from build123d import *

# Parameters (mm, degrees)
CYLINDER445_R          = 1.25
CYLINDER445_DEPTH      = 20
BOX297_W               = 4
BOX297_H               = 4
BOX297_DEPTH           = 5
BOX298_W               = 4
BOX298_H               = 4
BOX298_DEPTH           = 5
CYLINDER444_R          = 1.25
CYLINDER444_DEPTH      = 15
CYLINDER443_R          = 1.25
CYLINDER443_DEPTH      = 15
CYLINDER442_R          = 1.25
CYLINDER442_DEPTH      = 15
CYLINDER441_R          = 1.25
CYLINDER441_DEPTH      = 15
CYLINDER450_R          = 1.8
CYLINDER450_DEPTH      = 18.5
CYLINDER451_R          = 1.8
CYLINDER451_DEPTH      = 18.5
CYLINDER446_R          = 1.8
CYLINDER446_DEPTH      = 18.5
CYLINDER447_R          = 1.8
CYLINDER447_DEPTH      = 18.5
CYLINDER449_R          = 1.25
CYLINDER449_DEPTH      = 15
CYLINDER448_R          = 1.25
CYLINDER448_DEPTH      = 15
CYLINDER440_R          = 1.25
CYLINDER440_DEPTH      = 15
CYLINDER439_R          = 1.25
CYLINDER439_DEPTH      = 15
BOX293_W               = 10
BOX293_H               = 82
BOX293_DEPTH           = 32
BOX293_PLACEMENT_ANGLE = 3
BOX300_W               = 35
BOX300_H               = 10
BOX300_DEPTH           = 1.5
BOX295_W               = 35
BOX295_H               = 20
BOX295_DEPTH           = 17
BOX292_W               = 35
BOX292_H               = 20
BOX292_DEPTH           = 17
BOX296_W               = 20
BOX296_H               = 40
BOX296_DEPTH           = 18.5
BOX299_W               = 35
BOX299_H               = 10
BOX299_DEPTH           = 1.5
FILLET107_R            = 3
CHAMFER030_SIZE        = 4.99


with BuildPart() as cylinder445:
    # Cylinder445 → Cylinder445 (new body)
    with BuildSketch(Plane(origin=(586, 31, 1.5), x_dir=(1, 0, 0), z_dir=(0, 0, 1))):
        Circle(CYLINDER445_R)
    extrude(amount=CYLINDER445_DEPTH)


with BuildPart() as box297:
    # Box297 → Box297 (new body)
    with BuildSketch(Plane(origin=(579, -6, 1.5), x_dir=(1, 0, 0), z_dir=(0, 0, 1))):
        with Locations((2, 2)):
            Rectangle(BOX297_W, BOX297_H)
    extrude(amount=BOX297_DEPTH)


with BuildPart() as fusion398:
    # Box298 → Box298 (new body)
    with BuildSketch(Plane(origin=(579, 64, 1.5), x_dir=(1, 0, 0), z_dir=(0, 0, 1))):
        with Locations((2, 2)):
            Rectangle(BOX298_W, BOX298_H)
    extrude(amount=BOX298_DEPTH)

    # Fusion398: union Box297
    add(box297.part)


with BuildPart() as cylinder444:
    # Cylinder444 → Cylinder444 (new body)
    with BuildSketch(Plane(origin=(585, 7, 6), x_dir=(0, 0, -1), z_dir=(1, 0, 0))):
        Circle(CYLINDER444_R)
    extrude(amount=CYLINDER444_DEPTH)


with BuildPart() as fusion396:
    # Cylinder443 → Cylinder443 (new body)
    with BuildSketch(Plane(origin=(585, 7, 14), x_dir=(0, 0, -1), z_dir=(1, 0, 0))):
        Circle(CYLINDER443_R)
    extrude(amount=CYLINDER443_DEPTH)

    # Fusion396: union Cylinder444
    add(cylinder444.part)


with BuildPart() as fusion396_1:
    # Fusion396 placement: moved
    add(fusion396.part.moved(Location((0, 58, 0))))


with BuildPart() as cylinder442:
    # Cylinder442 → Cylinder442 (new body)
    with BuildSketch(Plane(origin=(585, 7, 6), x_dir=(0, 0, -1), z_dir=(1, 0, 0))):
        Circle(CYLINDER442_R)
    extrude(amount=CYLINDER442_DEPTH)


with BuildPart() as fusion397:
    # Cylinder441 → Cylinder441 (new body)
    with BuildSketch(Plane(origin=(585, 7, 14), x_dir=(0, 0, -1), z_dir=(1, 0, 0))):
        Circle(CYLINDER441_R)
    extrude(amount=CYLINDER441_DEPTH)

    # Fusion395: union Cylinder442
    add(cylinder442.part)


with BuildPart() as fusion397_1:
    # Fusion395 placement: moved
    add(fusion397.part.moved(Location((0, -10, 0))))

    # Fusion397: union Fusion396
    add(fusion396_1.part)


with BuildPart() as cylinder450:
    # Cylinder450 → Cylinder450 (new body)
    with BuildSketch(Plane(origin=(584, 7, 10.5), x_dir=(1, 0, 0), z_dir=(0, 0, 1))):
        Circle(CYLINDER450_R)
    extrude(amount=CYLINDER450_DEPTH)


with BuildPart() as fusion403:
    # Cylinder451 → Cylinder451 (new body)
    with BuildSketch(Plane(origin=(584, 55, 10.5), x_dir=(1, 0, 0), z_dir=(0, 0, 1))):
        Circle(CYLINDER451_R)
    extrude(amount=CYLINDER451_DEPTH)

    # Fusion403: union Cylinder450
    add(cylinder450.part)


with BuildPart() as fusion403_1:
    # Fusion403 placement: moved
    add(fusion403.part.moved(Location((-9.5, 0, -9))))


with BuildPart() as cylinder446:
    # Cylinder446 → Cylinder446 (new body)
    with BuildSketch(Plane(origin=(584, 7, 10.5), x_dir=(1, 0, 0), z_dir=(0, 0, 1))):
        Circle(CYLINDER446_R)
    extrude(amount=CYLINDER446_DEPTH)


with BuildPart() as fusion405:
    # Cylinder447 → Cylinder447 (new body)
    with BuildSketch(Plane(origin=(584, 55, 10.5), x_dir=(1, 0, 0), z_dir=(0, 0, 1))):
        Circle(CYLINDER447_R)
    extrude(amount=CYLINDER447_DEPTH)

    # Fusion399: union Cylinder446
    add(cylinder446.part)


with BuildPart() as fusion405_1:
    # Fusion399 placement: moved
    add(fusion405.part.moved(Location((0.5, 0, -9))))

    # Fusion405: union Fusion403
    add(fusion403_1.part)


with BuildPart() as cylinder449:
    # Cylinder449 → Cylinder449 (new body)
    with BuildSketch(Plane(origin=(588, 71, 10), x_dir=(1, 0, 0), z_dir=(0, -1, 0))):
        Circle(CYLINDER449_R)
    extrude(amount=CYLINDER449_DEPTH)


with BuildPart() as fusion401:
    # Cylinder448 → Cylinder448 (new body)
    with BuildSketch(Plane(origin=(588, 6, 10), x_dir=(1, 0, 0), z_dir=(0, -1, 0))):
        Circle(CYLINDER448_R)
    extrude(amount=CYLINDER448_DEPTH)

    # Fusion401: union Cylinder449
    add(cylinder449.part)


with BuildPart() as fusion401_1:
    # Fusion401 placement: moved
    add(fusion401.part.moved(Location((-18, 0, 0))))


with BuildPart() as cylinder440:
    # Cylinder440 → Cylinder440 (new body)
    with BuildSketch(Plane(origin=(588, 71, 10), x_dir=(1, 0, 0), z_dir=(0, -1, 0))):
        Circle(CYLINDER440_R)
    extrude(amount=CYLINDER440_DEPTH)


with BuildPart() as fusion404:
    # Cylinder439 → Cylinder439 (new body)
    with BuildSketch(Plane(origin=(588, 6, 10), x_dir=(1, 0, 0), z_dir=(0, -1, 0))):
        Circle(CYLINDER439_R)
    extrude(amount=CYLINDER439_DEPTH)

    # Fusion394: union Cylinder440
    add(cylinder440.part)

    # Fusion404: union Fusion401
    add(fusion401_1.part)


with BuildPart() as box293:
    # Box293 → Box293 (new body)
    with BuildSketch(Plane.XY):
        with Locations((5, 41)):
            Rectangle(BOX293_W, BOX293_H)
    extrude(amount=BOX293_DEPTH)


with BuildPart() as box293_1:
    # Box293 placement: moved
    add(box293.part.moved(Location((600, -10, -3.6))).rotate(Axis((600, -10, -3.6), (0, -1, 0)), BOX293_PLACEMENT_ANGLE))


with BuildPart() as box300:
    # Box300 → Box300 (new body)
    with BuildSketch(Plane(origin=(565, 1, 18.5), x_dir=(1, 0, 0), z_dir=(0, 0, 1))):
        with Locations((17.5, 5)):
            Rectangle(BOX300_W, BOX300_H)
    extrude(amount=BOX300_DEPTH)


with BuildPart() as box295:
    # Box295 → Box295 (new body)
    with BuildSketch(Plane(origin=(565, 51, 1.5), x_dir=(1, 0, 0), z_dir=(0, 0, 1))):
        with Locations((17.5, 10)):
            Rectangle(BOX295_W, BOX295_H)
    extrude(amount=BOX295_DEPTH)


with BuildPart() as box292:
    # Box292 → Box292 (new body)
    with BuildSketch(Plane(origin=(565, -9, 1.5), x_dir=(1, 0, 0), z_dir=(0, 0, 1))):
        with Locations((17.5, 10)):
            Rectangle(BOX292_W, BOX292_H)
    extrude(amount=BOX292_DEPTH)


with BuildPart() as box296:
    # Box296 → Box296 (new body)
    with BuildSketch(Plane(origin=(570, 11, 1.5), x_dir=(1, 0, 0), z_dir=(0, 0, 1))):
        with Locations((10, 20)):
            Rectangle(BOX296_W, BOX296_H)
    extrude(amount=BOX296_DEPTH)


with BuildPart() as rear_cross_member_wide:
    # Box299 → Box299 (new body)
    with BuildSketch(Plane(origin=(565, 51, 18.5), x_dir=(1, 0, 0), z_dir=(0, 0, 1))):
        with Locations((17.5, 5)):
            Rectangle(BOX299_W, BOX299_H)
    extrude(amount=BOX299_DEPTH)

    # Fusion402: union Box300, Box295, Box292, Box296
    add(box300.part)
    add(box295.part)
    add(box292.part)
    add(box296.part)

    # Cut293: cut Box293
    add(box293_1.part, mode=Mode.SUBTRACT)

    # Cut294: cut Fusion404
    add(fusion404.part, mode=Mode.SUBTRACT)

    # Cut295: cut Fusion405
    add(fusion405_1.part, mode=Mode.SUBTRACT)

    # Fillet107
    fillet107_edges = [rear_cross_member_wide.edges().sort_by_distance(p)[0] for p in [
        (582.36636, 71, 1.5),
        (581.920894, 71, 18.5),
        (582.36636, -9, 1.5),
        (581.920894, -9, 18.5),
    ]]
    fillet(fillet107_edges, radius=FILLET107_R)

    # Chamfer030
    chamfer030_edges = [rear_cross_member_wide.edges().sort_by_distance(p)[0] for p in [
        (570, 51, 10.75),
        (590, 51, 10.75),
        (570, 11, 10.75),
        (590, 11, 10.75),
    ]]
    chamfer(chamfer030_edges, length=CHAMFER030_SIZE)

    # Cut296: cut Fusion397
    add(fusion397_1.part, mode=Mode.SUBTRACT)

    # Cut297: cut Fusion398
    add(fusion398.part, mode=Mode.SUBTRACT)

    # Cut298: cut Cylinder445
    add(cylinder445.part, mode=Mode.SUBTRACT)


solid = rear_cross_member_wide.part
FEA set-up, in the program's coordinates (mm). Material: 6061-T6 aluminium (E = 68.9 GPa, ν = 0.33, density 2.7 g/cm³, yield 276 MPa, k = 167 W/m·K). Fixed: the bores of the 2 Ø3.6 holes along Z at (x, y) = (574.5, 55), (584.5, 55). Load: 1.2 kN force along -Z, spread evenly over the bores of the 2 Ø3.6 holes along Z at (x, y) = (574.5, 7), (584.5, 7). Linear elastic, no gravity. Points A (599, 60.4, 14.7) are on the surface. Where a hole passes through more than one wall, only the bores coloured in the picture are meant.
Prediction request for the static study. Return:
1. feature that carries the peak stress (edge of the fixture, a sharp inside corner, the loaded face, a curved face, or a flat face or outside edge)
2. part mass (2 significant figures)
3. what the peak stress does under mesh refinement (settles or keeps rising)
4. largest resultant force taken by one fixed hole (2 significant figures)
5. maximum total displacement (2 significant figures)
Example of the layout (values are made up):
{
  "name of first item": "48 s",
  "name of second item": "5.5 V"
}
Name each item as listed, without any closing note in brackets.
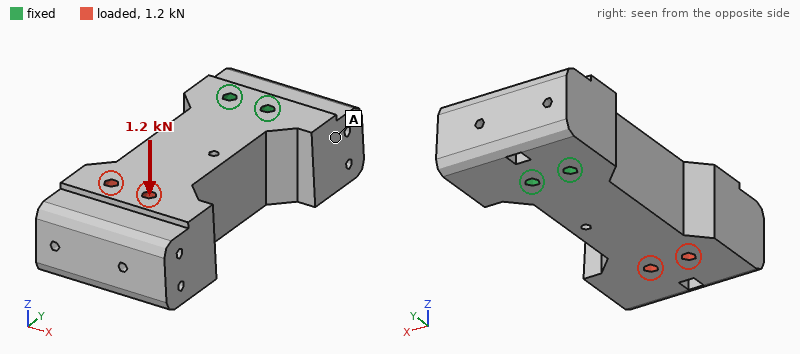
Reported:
{
  "feature that carries the peak stress": "edge of the fixture",
  "part mass": "100 g",
  "what the peak stress does under mesh refinement": "keeps rising",
  "largest resultant force taken by one fixed hole": "600 N",
  "maximum total displacement": "94 µm"
}
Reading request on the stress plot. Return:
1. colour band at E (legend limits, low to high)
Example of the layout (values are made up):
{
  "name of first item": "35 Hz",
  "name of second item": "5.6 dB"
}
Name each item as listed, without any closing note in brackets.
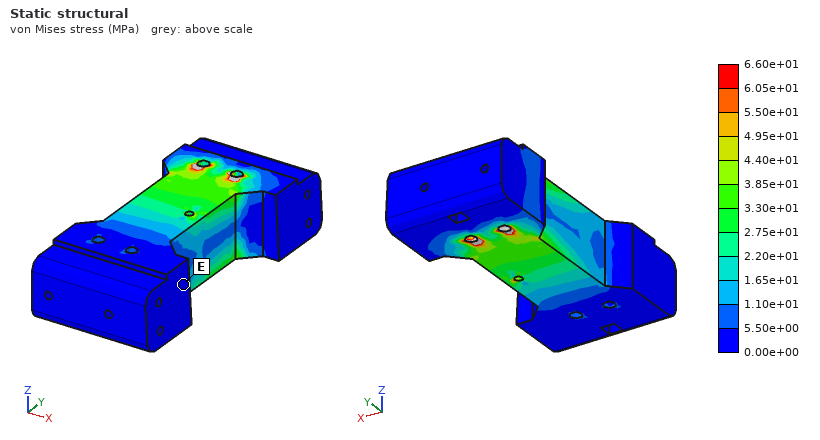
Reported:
{
  "colour band at E": "0.00e+00 to 5.50e+00 MPa"
}
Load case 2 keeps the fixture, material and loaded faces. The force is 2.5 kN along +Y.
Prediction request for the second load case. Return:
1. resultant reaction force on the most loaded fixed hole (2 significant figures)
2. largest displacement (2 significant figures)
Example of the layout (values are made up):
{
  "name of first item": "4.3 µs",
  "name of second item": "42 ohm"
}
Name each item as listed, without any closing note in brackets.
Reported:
{
  "resultant reaction force on the most loaded fixed hole": "1.3 kN",
  "largest displacement": "5.4 µm"
}
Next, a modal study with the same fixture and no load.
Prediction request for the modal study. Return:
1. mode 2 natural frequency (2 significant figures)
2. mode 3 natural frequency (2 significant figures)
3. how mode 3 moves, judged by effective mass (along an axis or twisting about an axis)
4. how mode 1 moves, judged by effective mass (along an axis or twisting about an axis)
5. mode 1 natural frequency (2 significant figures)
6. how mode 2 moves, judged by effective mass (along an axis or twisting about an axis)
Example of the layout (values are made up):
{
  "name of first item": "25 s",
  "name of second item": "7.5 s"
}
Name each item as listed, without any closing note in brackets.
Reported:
{
  "mode 2 natural frequency": "3100 Hz",
  "mode 3 natural frequency": "7700 Hz",
  "how mode 3 moves, judged by effective mass": "twisting about Y",
  "how mode 1 moves, judged by effective mass": "along Z",
  "mode 1 natural frequency": "3000 Hz",
  "how mode 2 moves, judged by effective mass": "along X"
}
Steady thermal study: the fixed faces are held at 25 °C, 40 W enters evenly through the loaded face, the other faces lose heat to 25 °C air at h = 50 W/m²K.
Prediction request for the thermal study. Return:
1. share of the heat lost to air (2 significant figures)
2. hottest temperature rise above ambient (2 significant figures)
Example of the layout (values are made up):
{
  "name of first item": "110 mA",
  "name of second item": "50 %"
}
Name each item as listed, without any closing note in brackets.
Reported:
{
  "share of the heat lost to air": "16 %",
  "hottest temperature rise above ambient": "27 K"
}
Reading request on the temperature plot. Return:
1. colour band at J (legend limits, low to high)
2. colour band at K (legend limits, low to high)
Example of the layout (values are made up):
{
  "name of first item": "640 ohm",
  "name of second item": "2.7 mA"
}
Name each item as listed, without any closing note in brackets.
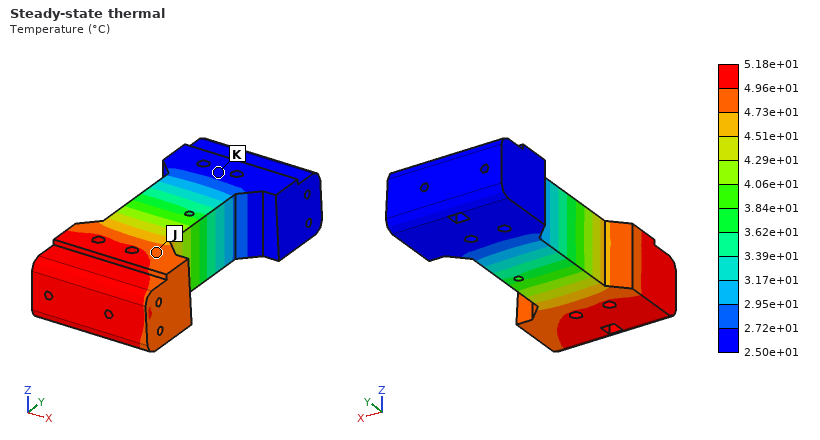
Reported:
{
  "colour band at J": "4.73e+01 to 4.96e+01 °C",
  "colour band at K": "2.50e+01 to 2.72e+01 °C"
}
